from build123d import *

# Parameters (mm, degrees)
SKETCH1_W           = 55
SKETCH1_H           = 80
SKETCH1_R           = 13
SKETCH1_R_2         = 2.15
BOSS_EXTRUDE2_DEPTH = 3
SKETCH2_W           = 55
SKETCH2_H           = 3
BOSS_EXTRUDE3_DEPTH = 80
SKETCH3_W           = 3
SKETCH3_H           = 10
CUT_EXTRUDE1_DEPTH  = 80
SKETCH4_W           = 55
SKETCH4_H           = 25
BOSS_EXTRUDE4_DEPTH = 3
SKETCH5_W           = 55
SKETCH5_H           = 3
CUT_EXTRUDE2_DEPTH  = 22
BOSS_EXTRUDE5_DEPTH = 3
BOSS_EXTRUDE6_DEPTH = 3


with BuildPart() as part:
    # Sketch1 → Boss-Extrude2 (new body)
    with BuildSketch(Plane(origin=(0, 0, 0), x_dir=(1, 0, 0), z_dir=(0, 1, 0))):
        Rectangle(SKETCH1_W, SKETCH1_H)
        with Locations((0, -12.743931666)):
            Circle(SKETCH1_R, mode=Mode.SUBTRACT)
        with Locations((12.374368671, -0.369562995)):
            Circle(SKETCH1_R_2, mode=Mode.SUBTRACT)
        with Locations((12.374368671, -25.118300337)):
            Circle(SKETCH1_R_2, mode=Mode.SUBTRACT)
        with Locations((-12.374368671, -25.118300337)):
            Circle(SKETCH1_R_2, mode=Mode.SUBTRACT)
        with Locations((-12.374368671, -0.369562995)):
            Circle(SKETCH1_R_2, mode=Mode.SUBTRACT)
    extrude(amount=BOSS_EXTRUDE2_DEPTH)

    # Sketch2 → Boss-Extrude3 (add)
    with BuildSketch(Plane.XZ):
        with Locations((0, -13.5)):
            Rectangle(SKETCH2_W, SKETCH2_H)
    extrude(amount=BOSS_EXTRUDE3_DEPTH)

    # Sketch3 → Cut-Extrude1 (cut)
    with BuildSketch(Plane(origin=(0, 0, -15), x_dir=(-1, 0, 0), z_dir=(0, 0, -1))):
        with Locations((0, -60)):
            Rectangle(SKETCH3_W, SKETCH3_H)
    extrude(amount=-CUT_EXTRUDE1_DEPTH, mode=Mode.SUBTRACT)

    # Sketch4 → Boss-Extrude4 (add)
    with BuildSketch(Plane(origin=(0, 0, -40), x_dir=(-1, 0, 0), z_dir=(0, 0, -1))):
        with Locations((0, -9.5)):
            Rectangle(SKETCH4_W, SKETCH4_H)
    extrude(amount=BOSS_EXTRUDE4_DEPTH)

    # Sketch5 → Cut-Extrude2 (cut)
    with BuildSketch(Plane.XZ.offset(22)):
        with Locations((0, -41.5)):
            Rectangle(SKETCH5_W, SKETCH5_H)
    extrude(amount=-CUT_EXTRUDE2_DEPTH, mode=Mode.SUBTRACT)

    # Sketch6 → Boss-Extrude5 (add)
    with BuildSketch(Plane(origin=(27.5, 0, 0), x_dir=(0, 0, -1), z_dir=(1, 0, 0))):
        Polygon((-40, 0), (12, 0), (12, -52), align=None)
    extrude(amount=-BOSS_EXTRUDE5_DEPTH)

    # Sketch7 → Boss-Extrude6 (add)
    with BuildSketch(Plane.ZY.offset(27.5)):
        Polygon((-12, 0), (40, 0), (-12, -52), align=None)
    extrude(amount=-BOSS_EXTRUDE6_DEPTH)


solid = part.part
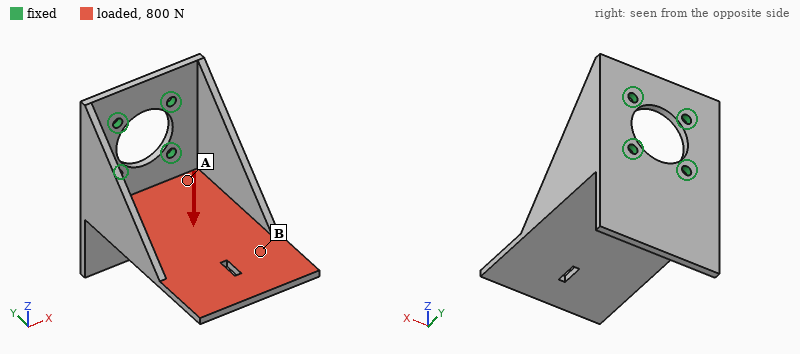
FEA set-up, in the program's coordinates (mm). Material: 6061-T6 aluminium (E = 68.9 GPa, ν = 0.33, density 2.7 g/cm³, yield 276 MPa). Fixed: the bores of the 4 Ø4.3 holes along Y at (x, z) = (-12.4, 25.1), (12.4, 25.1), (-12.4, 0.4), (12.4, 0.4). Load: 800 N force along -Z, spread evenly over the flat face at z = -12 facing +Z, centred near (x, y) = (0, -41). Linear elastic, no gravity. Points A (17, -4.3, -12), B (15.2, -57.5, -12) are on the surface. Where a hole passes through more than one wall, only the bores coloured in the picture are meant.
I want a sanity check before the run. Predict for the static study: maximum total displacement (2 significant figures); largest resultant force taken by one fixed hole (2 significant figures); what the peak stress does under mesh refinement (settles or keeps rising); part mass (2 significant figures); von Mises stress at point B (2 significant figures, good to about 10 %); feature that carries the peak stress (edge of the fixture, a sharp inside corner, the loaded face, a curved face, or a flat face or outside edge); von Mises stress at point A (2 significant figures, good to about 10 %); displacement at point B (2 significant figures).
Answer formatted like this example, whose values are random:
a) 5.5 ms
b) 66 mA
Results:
a) 0.77 mm
b) 570 N
c) keeps rising
d) 90 g
e) 46 MPa
f) edge of the fixture
g) 20 MPa
h) 0.38 mm
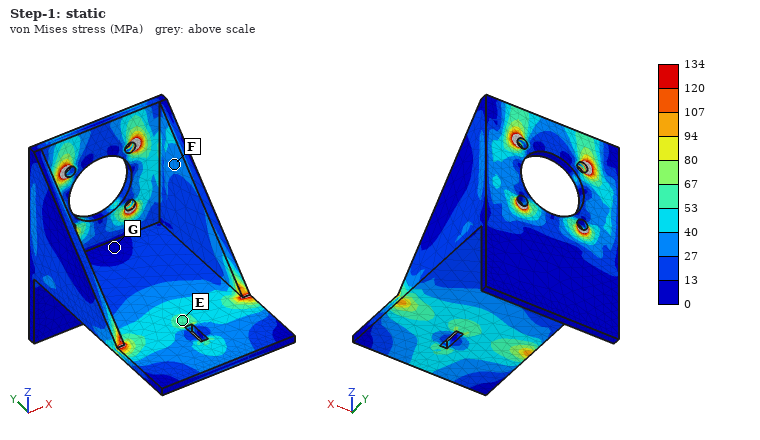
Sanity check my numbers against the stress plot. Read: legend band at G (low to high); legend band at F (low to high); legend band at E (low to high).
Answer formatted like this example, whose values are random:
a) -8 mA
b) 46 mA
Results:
a) 0 to 13 MPa
b) 27 to 40 MPa
c) 53 to 67 MPa
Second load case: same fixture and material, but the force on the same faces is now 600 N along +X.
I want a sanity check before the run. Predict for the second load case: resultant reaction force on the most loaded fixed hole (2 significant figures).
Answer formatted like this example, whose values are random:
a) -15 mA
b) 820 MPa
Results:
a) 900 N
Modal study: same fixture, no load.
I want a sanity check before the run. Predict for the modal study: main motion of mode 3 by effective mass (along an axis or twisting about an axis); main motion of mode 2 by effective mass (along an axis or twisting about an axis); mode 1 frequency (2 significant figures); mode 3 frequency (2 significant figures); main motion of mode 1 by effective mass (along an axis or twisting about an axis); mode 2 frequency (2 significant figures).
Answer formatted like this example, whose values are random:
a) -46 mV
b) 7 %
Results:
a) along Y
b) along X
c) 1100 Hz
d) 2000 Hz
e) along Z
f) 1200 Hz
